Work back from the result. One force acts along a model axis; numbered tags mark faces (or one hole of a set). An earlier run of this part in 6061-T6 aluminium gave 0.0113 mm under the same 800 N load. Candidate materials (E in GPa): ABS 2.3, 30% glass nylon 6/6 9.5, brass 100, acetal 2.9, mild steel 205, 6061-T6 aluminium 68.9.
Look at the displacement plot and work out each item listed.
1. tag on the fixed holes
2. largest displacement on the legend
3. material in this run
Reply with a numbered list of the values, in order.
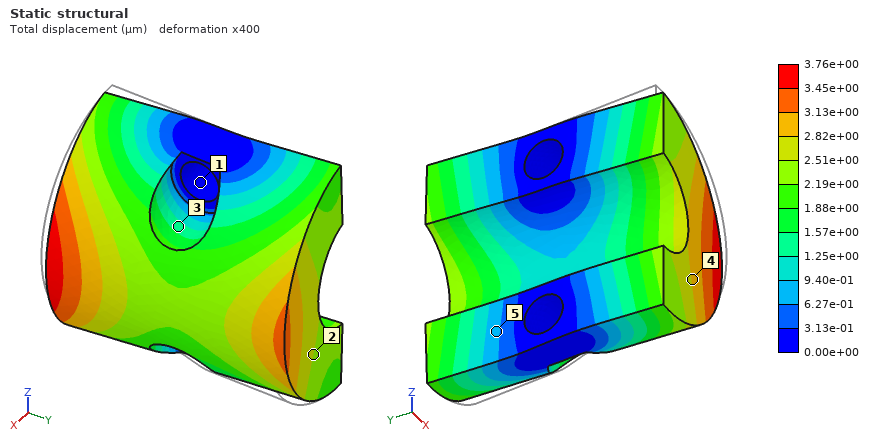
1. 1
2. 3.76e+00 µm
3. mild steel
